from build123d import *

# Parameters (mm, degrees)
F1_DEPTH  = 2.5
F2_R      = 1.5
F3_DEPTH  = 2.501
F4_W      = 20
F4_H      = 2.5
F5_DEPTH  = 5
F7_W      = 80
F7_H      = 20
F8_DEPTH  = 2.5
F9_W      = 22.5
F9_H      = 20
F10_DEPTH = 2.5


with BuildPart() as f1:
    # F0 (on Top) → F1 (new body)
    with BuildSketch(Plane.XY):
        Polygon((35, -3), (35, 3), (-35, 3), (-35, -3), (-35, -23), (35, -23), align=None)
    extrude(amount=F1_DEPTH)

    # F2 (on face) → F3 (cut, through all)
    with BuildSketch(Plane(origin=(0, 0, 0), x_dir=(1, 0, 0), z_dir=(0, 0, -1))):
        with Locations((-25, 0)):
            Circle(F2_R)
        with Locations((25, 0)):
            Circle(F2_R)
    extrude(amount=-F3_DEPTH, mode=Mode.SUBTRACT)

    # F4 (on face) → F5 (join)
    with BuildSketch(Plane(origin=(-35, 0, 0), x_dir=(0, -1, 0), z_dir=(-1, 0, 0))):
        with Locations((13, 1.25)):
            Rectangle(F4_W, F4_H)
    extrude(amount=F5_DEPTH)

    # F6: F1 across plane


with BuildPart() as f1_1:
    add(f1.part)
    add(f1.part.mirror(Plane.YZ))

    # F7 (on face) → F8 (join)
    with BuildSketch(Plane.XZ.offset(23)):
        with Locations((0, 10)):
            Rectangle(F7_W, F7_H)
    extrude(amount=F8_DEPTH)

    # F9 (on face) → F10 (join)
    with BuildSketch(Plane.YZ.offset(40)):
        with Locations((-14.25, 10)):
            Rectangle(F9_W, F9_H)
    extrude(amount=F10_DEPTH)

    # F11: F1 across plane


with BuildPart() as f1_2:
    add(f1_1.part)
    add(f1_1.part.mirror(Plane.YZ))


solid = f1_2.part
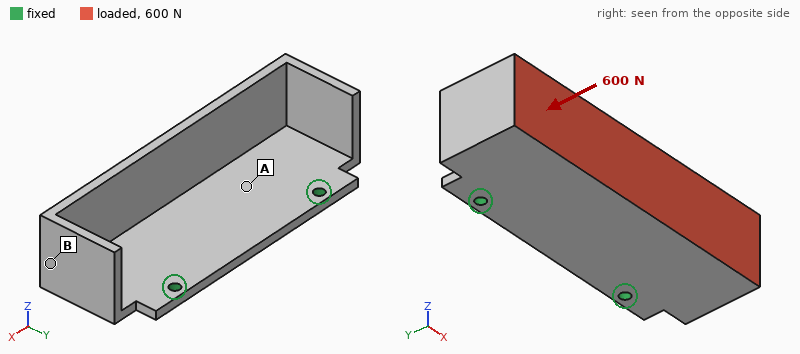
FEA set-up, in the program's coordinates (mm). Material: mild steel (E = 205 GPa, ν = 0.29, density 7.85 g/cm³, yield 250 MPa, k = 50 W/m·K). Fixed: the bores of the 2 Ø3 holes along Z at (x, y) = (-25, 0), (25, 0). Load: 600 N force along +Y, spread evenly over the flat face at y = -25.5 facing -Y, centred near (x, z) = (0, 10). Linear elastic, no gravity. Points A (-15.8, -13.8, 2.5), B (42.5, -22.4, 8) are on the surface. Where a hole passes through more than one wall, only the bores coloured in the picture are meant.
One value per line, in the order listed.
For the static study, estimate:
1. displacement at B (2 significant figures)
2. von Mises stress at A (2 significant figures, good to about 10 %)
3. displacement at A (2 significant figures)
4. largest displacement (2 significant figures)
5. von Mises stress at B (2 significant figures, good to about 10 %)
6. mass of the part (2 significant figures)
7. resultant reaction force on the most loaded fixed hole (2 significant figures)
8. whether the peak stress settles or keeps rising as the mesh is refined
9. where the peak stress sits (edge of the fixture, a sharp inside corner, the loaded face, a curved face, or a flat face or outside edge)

0.097 mm
45 MPa
0.043 mm
0.17 mm
19 MPa
88 g
300 N
keeps rising
edge of the fixture
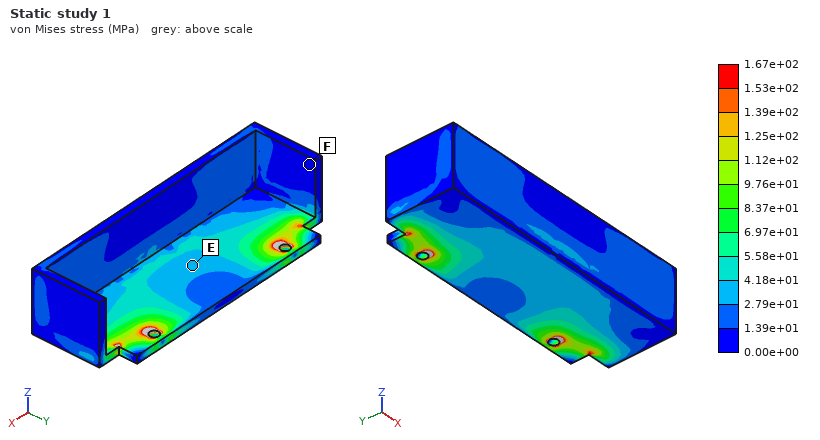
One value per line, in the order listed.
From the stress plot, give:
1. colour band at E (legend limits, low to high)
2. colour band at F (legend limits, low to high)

2.79e+01 to 4.18e+01 MPa
0.00e+00 to 1.39e+01 MPa
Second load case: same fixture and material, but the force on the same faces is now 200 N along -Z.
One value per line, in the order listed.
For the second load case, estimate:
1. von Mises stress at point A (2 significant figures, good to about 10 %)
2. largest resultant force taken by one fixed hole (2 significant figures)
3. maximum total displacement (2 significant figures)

22 MPa
100 N
0.12 mm
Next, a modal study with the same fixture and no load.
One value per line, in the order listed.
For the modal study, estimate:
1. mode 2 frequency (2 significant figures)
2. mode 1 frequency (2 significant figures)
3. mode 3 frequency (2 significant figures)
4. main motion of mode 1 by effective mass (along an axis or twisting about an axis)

1500 Hz
1100 Hz
4000 Hz
along Z
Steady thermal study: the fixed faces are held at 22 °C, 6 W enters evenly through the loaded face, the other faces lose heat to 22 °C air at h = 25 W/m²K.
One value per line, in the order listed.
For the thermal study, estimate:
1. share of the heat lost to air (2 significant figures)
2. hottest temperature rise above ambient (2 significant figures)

37 %
18 K
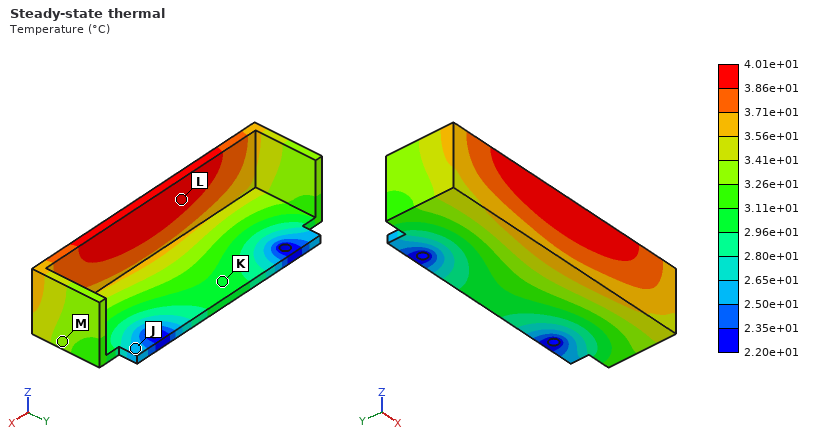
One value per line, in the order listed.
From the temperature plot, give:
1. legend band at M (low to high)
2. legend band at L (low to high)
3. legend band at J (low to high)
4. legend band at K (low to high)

3.26e+01 to 3.41e+01 °C
3.86e+01 to 4.01e+01 °C
2.50e+01 to 2.65e+01 °C
2.96e+01 to 3.11e+01 °C
